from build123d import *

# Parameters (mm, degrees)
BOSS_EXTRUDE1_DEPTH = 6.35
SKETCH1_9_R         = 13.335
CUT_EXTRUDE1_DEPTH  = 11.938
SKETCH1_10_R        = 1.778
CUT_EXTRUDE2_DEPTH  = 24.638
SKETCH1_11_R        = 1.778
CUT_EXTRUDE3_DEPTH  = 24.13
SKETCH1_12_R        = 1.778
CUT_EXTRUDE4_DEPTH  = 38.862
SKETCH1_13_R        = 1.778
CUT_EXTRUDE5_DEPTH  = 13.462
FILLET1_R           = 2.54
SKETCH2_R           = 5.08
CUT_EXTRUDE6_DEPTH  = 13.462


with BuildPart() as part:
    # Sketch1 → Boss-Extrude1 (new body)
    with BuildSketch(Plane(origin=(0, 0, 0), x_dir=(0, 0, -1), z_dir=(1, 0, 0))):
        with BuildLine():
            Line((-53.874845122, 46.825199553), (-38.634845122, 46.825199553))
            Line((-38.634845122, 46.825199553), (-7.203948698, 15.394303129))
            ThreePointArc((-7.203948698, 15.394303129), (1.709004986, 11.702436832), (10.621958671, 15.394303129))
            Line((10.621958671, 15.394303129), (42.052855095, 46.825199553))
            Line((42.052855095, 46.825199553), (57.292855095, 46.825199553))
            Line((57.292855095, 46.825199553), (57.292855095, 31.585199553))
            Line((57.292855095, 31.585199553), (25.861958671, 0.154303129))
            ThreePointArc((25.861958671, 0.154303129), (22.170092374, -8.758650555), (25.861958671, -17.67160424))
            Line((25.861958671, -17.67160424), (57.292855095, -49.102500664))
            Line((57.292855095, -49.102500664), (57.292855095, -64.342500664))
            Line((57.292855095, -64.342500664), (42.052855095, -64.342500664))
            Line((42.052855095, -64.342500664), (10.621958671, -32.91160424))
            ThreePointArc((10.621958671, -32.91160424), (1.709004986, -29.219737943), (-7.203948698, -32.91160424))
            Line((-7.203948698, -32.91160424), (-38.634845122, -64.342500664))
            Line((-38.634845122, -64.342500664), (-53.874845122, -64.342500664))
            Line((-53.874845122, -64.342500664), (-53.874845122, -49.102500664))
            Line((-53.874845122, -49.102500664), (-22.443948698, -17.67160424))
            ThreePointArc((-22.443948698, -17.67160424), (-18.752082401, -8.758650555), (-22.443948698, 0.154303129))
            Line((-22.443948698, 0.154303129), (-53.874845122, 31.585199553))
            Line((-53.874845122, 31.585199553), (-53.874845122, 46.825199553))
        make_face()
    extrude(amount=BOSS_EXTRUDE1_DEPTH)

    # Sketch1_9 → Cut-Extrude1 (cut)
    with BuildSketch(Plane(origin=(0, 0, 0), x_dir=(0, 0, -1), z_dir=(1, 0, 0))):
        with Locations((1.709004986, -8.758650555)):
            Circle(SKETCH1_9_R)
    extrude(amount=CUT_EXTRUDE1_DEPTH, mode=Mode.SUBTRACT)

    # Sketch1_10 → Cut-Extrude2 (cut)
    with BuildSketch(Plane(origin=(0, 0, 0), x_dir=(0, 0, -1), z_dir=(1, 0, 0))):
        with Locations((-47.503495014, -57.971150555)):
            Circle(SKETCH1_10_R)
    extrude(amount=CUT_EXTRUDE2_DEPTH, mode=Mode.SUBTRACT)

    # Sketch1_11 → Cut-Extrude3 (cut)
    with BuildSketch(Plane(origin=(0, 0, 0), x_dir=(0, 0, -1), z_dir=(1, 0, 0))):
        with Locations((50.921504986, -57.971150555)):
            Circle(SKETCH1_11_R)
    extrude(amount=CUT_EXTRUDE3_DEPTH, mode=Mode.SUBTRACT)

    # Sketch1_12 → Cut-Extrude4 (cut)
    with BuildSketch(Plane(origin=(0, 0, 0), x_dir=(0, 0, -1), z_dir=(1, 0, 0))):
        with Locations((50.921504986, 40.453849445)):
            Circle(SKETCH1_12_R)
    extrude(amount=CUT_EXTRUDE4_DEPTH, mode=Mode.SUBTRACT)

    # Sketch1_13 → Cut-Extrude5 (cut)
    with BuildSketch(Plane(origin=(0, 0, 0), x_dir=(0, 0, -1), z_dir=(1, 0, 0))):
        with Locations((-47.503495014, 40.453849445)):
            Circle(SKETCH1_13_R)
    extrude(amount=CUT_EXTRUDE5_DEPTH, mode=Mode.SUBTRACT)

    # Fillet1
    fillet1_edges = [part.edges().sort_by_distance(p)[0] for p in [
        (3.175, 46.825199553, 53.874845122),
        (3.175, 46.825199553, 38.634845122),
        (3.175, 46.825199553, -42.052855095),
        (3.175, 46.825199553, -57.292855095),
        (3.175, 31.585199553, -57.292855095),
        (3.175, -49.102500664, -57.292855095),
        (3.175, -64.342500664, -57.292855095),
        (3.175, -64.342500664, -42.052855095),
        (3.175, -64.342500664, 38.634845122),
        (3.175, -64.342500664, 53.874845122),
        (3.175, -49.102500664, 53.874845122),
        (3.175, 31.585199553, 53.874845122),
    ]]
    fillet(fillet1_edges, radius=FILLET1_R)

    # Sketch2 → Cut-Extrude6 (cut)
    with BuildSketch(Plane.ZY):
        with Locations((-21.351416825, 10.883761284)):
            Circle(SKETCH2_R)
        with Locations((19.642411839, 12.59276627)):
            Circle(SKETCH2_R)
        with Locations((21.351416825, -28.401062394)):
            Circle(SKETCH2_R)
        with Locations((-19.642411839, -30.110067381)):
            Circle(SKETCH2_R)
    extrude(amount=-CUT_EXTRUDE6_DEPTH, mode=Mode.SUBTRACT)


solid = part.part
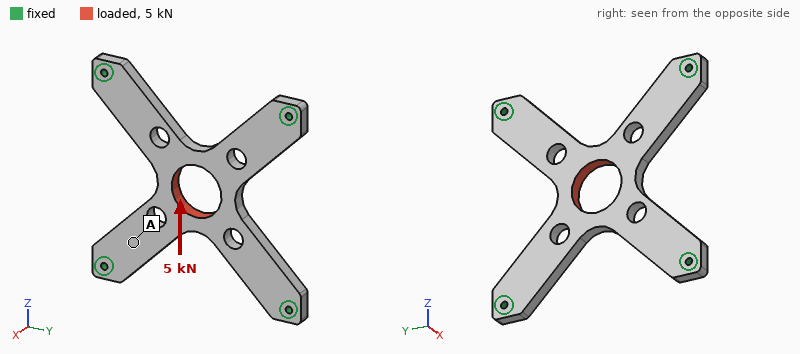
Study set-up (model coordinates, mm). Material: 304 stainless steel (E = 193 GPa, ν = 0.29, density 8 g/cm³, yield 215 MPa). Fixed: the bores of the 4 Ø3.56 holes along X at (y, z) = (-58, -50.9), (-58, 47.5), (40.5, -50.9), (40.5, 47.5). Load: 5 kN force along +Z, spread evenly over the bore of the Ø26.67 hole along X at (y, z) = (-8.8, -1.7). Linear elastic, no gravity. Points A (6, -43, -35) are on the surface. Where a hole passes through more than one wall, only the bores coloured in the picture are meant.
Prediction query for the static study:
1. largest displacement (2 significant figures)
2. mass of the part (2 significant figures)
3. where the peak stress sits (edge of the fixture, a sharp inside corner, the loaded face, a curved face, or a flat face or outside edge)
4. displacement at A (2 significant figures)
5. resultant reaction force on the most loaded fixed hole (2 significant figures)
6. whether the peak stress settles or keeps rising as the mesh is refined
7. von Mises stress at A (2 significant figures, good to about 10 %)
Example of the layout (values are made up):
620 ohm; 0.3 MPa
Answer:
9.0 µm; 260 g; edge of the fixture; 2.9 µm; 1.7 kN; keeps rising; 11 MPa
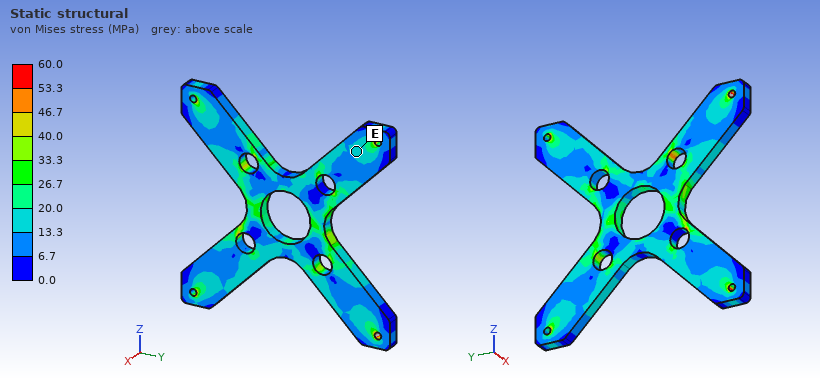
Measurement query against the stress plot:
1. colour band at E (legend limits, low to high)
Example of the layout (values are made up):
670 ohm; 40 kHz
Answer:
13.3 to 20.0 MPa
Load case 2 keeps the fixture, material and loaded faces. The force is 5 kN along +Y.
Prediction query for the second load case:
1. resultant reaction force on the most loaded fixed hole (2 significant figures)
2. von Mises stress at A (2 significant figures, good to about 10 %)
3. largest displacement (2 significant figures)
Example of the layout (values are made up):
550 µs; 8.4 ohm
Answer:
1.7 kN; 12 MPa; 8.7 µm
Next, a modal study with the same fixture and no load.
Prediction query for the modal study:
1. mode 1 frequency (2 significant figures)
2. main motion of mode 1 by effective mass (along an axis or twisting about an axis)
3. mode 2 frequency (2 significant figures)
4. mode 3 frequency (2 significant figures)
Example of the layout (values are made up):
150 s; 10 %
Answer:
1900 Hz; along X; 4200 Hz; 4200 Hz
